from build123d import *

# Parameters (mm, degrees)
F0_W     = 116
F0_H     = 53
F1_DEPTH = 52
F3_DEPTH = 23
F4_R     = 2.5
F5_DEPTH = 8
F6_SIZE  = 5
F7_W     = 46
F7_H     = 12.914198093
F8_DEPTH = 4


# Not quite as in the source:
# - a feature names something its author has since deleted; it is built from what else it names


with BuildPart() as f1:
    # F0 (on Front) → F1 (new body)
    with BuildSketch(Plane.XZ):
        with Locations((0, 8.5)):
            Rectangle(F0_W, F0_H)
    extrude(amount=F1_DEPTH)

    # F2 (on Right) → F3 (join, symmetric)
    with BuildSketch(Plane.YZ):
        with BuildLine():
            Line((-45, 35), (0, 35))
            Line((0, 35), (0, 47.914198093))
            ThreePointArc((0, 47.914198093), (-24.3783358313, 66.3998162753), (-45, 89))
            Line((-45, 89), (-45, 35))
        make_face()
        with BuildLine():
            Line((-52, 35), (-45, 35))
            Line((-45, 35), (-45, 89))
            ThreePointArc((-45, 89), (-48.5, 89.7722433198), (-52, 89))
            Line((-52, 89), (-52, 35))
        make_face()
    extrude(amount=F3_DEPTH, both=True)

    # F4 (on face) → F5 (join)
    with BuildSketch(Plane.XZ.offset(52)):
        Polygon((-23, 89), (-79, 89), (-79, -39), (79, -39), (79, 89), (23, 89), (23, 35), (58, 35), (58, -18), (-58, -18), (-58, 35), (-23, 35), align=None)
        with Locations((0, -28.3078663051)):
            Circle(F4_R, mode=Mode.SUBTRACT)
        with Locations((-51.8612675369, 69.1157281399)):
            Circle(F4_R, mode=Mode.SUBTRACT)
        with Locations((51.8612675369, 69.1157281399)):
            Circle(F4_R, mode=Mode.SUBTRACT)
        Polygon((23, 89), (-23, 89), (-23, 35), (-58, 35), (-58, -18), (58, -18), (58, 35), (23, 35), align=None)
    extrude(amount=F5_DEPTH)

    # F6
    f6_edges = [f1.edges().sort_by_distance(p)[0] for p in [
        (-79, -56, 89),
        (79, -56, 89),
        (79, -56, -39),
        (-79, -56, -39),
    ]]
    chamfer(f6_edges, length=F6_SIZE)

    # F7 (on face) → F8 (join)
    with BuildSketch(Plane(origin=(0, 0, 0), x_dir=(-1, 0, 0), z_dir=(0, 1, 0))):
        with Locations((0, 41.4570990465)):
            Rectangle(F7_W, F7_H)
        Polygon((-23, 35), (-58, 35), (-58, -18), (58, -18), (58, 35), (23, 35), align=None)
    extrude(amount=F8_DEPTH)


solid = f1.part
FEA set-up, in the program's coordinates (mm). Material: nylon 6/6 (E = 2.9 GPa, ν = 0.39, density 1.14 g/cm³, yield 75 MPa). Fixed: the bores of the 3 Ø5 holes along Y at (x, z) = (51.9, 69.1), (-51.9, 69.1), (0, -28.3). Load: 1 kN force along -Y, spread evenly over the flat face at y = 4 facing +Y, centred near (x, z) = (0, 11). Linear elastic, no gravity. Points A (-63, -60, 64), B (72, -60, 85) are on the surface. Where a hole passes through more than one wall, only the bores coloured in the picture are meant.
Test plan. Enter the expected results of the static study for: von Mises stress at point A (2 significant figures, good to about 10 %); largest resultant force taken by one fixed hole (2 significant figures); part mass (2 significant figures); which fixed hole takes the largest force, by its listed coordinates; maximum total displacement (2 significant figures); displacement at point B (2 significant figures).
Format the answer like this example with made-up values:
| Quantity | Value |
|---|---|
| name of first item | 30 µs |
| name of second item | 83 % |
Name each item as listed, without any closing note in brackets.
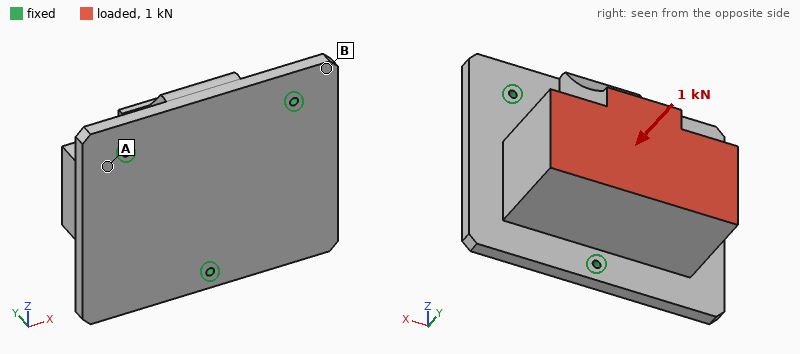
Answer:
| Quantity | Value |
|---|---|
| von Mises stress at point A | 1.4 MPa |
| largest resultant force taken by one fixed hole | 620 N |
| part mass | 670 g |
| which fixed hole takes the largest force, by its listed coordinates | (0, -28.3) |
| maximum total displacement | 0.11 mm |
| displacement at point B | 0.045 mm |
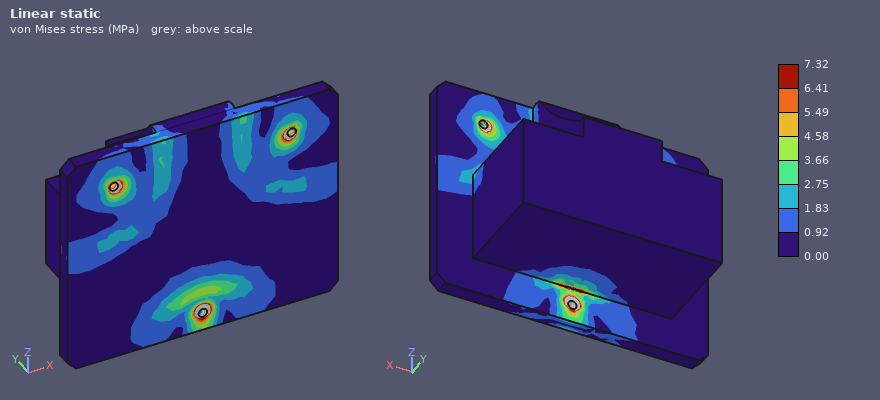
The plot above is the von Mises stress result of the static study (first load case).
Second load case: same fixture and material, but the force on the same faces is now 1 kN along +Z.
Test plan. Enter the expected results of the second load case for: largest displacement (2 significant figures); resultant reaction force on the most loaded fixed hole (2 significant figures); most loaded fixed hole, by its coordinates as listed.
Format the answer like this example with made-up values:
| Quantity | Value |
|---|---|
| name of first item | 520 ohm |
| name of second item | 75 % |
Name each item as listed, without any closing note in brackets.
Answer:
| Quantity | Value |
|---|---|
| largest displacement | 0.25 mm |
| resultant reaction force on the most loaded fixed hole | 830 N |
| most loaded fixed hole, by its coordinates as listed | (0, -28.3) |
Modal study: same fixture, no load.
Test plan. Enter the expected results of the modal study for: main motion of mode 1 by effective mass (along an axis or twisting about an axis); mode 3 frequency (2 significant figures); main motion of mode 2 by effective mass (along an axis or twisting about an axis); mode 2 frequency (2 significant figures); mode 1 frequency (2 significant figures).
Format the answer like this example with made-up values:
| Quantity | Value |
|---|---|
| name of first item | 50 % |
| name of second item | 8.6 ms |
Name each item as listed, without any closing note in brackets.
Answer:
| Quantity | Value |
|---|---|
| main motion of mode 1 by effective mass | along X |
| mode 3 frequency | 740 Hz |
| main motion of mode 2 by effective mass | along Y |
| mode 2 frequency | 590 Hz |
| mode 1 frequency | 400 Hz |
